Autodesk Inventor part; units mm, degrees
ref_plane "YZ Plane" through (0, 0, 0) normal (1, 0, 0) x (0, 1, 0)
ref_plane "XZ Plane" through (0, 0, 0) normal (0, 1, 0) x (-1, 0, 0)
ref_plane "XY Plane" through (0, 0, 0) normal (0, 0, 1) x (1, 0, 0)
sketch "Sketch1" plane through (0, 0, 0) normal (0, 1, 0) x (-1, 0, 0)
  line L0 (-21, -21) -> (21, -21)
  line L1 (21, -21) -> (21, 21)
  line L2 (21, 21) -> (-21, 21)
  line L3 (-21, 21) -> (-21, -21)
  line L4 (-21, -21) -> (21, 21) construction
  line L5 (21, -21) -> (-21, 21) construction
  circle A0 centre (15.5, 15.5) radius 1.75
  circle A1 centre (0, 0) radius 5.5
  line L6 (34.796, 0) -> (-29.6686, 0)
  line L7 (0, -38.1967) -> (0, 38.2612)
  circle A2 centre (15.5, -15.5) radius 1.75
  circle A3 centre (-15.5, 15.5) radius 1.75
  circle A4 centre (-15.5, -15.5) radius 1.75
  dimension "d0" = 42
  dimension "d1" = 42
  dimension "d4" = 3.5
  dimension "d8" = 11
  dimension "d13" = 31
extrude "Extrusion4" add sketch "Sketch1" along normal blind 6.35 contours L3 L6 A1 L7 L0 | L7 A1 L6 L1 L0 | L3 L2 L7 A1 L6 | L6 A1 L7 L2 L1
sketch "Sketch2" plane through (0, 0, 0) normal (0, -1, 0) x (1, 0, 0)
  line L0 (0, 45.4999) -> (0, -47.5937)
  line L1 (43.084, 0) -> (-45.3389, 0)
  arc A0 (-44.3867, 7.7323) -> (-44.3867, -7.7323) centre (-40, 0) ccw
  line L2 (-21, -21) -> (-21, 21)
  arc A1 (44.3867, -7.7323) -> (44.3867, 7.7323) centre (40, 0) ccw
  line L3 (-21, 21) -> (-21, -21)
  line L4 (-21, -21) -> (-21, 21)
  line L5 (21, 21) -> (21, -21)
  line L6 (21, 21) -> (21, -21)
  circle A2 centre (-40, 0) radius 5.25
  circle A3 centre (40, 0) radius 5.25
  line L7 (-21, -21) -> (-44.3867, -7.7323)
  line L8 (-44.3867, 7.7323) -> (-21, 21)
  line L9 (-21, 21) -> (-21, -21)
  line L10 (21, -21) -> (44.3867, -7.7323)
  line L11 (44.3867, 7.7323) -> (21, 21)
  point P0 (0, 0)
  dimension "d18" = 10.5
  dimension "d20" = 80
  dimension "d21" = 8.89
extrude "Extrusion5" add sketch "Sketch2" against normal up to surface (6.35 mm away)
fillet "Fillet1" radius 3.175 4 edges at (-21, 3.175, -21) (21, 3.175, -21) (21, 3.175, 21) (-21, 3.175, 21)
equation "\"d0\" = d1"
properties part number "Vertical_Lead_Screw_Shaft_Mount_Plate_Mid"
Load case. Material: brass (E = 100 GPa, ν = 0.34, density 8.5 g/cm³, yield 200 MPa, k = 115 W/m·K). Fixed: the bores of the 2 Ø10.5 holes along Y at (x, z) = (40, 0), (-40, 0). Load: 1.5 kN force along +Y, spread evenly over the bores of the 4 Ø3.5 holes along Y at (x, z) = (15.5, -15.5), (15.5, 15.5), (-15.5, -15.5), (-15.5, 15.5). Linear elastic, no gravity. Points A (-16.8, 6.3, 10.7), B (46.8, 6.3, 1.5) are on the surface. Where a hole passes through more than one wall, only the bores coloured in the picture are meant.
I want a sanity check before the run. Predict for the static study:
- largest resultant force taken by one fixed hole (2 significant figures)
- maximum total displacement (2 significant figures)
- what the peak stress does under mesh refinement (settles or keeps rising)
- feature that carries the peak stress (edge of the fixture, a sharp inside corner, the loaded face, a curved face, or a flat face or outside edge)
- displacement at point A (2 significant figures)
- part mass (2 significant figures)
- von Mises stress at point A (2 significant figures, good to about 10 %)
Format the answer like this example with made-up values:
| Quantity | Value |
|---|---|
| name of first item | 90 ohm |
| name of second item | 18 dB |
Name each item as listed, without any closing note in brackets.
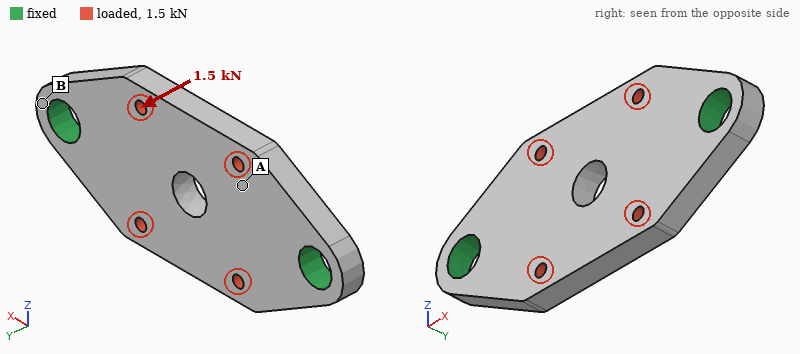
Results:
| Quantity | Value |
|---|---|
| largest resultant force taken by one fixed hole | 750 N |
| maximum total displacement | 41 µm |
| what the peak stress does under mesh refinement | keeps rising |
| feature that carries the peak stress | edge of the fixture |
| displacement at point A | 25 µm |
| part mass | 160 g |
| von Mises stress at point A | 20 MPa |
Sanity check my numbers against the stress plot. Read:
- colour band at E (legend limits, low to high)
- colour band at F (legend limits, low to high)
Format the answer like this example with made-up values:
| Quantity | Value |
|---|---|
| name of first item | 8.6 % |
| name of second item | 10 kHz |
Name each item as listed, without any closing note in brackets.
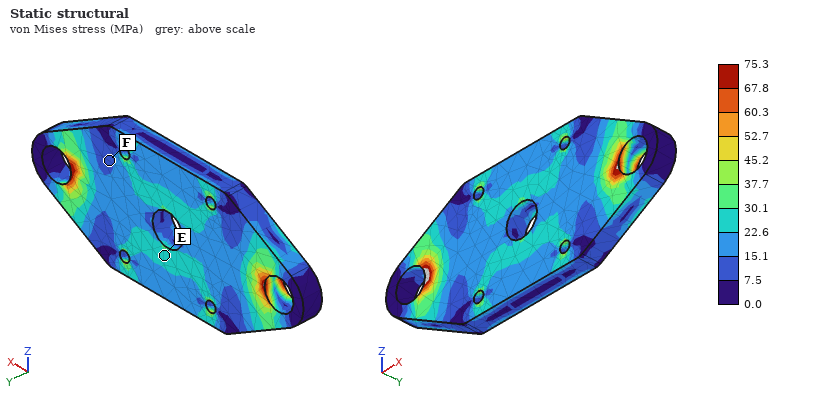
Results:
| Quantity | Value |
|---|---|
| colour band at E | 22.6 to 30.1 MPa |
| colour band at F | 7.5 to 15.1 MPa |
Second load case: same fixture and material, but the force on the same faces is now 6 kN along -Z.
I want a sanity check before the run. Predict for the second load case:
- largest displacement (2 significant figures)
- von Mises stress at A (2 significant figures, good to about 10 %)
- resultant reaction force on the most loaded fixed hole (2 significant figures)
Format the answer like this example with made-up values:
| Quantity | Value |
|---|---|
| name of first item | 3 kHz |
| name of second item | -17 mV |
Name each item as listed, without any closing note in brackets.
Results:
| Quantity | Value |
|---|---|
| largest displacement | 16 µm |
| von Mises stress at A | 24 MPa |
| resultant reaction force on the most loaded fixed hole | 3.0 kN |
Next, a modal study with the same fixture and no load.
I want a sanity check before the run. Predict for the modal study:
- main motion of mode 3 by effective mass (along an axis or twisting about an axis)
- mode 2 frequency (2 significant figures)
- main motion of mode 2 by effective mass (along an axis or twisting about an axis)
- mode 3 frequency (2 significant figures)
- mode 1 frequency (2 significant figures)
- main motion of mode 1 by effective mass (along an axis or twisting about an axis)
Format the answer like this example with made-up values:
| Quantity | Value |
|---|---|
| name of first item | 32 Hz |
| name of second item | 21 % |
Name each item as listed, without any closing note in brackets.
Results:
| Quantity | Value |
|---|---|
| main motion of mode 3 by effective mass | twisting about Z |
| mode 2 frequency | 3900 Hz |
| main motion of mode 2 by effective mass | twisting about X |
| mode 3 frequency | 8600 Hz |
| mode 1 frequency | 3400 Hz |
| main motion of mode 1 by effective mass | along Y |
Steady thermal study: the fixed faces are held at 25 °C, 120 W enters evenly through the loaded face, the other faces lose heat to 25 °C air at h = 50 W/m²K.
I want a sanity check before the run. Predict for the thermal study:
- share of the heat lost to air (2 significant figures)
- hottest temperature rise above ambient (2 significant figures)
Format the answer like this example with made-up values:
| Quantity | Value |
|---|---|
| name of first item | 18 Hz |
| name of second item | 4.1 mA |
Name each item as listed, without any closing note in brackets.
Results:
| Quantity | Value |
|---|---|
| share of the heat lost to air | 12 % |
| hottest temperature rise above ambient | 64 K |
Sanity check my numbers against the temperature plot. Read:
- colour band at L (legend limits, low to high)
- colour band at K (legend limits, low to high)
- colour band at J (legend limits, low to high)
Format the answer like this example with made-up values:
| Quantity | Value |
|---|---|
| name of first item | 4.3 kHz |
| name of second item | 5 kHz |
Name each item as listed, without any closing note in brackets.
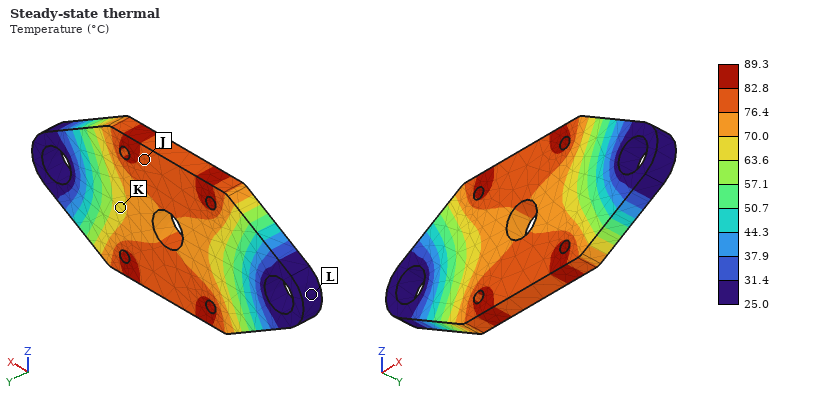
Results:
| Quantity | Value |
|---|---|
| colour band at L | 25.0 to 31.4 °C |
| colour band at K | 63.6 to 70.0 °C |
| colour band at J | 76.4 to 82.8 °C |
